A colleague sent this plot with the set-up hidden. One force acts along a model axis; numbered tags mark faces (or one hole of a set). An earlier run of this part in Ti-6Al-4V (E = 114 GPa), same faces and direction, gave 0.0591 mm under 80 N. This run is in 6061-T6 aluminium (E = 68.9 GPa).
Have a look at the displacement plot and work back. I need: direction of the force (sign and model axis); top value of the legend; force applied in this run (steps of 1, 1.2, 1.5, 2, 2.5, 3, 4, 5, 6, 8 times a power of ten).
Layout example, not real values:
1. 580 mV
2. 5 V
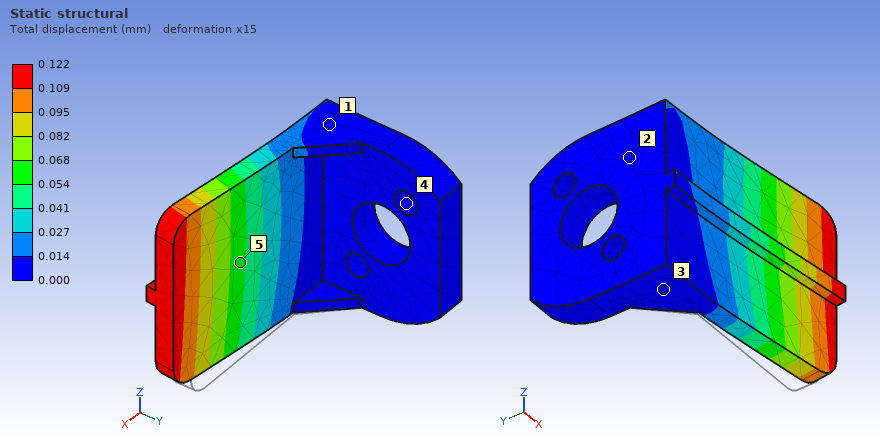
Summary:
1. -Y
2. 0.122 mm
3. 100 N
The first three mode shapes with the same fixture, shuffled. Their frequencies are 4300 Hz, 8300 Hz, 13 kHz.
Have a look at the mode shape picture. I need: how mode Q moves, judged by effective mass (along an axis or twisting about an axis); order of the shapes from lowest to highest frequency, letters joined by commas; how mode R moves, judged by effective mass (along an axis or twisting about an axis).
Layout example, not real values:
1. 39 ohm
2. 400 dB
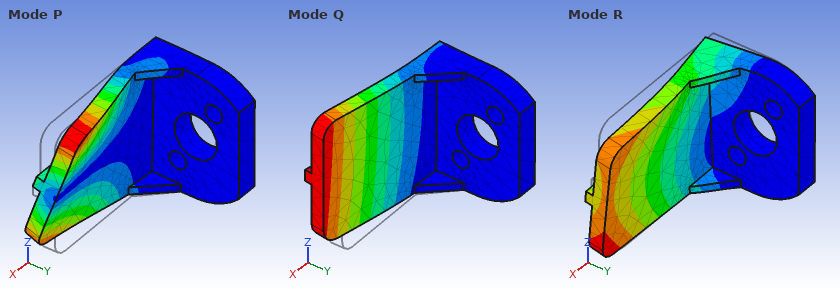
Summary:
1. along Y
2. Q, R, P
3. along Z
